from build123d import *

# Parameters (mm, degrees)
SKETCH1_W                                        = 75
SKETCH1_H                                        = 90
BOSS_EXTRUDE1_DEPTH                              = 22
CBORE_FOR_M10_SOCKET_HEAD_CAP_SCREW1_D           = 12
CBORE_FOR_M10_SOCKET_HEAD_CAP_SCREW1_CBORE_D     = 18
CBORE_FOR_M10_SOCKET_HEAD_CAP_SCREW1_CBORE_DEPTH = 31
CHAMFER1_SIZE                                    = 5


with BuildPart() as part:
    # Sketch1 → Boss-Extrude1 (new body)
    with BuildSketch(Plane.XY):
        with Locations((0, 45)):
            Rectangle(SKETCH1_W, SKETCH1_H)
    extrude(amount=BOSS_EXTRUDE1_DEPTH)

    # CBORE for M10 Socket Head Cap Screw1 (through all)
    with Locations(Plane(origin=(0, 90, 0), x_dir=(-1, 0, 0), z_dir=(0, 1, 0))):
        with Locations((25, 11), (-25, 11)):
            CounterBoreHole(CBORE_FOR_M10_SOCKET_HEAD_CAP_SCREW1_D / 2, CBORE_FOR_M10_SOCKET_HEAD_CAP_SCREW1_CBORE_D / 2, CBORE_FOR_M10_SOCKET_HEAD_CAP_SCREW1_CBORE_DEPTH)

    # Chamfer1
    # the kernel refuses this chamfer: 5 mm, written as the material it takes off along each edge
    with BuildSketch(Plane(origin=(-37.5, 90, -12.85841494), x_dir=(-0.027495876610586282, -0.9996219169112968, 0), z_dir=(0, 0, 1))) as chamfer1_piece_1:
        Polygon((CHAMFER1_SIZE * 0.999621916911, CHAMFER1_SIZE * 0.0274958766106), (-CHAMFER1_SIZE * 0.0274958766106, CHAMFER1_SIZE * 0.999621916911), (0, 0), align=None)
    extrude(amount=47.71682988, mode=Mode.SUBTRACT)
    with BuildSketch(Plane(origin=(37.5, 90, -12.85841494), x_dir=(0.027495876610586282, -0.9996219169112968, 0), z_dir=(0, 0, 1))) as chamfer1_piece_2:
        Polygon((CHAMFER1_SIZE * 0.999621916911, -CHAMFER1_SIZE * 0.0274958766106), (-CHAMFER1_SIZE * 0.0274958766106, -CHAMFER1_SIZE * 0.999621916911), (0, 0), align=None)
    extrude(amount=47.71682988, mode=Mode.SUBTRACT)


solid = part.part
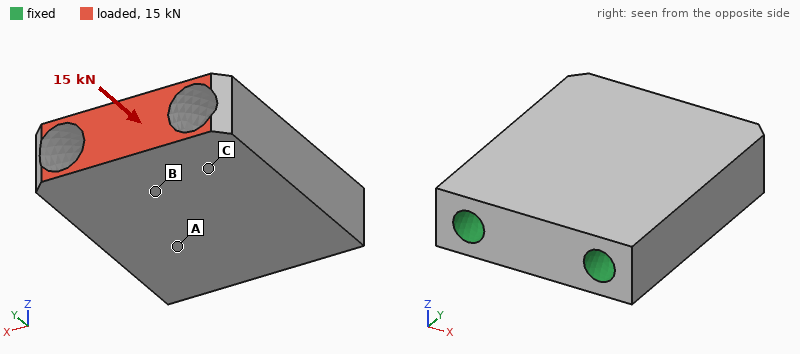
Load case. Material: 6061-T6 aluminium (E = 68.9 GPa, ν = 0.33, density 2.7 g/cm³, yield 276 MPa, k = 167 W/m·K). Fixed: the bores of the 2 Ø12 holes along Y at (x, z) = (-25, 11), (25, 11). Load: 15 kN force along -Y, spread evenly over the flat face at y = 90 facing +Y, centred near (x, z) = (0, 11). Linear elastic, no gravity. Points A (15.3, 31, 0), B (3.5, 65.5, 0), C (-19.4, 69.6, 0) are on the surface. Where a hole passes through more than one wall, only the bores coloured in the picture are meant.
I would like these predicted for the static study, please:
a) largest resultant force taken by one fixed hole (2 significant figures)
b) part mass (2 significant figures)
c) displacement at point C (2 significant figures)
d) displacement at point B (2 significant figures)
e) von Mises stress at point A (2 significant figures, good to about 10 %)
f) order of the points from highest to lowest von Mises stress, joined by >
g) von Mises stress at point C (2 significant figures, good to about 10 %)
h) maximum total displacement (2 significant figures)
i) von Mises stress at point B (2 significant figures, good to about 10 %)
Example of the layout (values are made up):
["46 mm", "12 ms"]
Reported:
["8.0 kN", "320 g", "5.3 µm", "5.5 µm", "4.9 MPa", "C > B > A", "18 MPa", "11 µm", "12 MPa"]
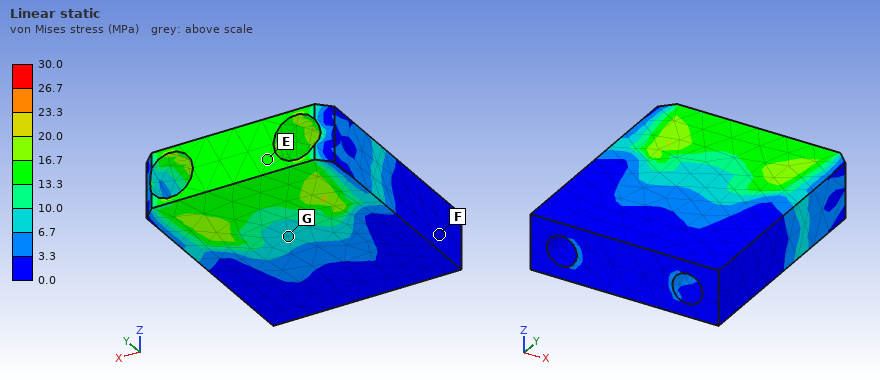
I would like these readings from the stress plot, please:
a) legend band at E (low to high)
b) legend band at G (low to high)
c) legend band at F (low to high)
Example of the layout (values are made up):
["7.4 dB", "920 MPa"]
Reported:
["13.3 to 16.7 MPa", "6.7 to 10.0 MPa", "0.0 to 3.3 MPa"]
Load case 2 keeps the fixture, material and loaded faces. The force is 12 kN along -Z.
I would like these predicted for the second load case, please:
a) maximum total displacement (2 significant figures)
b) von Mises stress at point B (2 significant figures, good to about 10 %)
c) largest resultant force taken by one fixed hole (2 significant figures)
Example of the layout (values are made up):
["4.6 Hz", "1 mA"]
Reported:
["0.13 mm", "61 MPa", "6.0 kN"]
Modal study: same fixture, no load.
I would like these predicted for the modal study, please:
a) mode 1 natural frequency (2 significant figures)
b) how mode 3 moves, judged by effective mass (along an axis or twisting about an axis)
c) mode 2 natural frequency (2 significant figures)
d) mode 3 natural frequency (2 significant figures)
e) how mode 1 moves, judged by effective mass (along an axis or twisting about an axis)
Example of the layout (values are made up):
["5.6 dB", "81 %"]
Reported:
["8500 Hz", "along X", "14 kHz", "16 kHz", "along Z"]
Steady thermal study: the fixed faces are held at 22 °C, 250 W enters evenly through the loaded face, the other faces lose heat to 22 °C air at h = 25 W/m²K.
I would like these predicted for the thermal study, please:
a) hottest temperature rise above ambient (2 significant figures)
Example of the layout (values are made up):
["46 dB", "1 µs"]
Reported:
["59 K"]
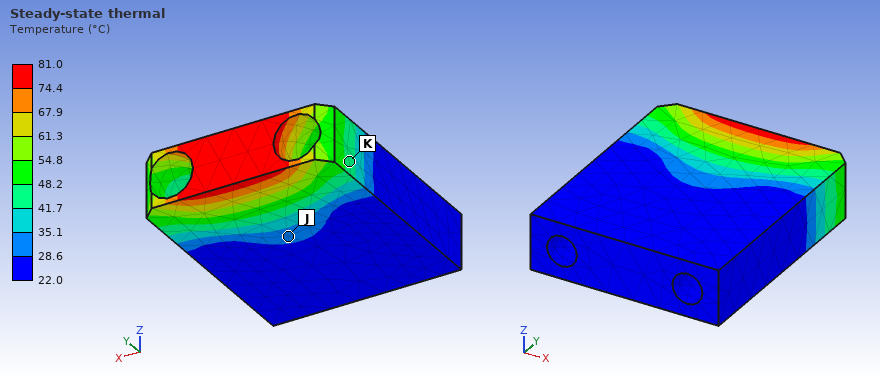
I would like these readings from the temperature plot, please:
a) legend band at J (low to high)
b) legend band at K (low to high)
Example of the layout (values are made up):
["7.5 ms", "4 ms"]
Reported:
["28.6 to 35.1 °C", "41.7 to 48.2 °C"]
